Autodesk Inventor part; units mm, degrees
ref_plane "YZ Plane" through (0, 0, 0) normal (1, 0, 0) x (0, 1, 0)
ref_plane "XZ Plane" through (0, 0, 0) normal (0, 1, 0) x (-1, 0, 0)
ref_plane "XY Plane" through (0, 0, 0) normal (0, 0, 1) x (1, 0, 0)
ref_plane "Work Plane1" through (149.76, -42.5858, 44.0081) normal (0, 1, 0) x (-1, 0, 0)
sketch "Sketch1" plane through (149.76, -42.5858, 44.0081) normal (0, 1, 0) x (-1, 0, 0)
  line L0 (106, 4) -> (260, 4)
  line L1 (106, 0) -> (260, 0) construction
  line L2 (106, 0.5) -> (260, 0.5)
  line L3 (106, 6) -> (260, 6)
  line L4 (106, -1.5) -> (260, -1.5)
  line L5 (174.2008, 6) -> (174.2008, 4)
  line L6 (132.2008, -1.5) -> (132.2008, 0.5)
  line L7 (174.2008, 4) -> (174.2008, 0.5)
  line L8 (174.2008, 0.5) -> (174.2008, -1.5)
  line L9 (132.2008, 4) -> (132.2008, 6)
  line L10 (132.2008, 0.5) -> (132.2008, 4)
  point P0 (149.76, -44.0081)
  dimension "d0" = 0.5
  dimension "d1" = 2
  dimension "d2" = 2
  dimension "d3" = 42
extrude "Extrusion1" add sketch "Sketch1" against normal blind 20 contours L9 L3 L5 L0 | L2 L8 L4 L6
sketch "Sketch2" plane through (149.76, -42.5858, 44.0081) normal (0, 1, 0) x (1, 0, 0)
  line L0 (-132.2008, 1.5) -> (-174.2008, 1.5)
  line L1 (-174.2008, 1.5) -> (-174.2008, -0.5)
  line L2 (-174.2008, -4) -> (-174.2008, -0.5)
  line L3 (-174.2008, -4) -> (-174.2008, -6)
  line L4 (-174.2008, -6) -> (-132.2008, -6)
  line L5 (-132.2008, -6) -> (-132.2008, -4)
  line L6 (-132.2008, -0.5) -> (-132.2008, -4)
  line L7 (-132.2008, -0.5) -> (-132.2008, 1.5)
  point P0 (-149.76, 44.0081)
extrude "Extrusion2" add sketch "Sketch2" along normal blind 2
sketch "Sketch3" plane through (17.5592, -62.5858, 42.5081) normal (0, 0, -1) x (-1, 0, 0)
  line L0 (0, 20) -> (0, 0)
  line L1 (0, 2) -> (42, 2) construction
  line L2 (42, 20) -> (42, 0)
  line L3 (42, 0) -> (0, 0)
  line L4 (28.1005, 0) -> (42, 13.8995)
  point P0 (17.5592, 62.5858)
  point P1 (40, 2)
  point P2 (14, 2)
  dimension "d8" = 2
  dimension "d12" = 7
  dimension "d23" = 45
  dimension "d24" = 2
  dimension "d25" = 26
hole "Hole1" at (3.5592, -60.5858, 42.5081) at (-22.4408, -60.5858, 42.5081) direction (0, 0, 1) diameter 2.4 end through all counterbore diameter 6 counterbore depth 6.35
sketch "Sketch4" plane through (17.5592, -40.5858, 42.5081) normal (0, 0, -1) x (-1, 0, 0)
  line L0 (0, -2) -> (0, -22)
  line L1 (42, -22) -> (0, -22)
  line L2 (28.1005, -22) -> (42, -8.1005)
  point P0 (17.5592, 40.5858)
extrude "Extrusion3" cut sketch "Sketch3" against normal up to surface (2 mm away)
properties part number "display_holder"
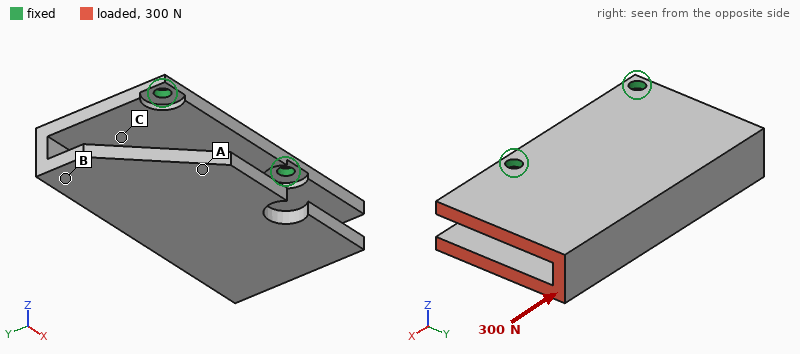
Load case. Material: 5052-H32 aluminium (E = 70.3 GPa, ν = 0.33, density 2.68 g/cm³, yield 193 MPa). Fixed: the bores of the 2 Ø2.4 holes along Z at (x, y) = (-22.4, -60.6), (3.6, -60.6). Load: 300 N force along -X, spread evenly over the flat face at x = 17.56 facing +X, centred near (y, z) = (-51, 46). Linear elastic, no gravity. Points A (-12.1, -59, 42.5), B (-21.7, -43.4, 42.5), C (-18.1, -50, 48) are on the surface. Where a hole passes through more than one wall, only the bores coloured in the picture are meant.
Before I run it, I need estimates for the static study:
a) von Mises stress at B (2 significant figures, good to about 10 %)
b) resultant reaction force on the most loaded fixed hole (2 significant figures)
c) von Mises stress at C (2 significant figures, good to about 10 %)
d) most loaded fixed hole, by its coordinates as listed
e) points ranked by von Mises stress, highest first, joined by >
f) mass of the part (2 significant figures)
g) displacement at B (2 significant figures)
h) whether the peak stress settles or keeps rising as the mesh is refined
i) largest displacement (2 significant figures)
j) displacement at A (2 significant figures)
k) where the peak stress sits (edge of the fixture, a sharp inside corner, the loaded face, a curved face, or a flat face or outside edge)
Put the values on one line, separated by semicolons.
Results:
17 MPa; 210 N; 30 MPa; (3.6, -60.6); C > B > A; 9.9 g; 0.073 mm; keeps rising; 0.10 mm; 0.050 mm; edge of the fixture
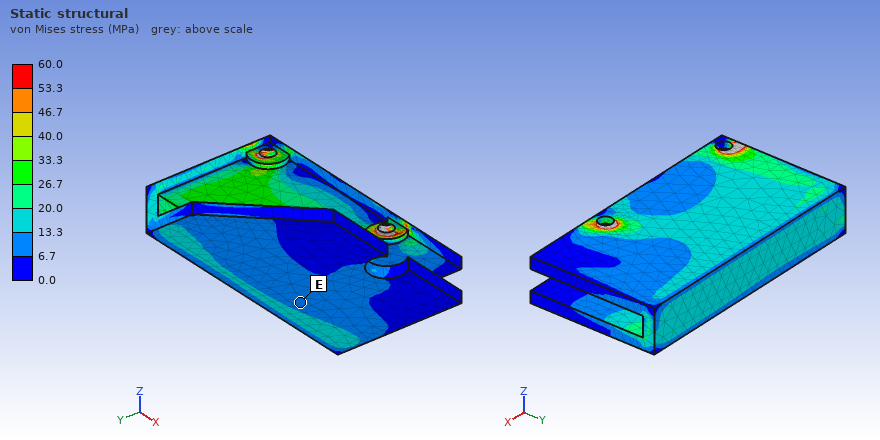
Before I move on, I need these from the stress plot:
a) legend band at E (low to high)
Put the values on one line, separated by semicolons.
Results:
6.7 to 13.3 MPa
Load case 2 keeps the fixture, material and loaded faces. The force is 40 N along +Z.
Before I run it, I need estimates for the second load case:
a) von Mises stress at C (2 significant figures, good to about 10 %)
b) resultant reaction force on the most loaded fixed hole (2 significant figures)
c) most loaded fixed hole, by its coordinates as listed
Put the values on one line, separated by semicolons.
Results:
15 MPa; 58 N; (3.6, -60.6)
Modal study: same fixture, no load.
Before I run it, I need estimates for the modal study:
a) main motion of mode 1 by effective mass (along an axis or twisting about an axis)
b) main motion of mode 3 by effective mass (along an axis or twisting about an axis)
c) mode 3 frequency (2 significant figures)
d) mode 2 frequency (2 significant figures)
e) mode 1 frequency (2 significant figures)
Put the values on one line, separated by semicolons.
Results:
along Z; along Z; 2700 Hz; 2200 Hz; 1300 Hz
